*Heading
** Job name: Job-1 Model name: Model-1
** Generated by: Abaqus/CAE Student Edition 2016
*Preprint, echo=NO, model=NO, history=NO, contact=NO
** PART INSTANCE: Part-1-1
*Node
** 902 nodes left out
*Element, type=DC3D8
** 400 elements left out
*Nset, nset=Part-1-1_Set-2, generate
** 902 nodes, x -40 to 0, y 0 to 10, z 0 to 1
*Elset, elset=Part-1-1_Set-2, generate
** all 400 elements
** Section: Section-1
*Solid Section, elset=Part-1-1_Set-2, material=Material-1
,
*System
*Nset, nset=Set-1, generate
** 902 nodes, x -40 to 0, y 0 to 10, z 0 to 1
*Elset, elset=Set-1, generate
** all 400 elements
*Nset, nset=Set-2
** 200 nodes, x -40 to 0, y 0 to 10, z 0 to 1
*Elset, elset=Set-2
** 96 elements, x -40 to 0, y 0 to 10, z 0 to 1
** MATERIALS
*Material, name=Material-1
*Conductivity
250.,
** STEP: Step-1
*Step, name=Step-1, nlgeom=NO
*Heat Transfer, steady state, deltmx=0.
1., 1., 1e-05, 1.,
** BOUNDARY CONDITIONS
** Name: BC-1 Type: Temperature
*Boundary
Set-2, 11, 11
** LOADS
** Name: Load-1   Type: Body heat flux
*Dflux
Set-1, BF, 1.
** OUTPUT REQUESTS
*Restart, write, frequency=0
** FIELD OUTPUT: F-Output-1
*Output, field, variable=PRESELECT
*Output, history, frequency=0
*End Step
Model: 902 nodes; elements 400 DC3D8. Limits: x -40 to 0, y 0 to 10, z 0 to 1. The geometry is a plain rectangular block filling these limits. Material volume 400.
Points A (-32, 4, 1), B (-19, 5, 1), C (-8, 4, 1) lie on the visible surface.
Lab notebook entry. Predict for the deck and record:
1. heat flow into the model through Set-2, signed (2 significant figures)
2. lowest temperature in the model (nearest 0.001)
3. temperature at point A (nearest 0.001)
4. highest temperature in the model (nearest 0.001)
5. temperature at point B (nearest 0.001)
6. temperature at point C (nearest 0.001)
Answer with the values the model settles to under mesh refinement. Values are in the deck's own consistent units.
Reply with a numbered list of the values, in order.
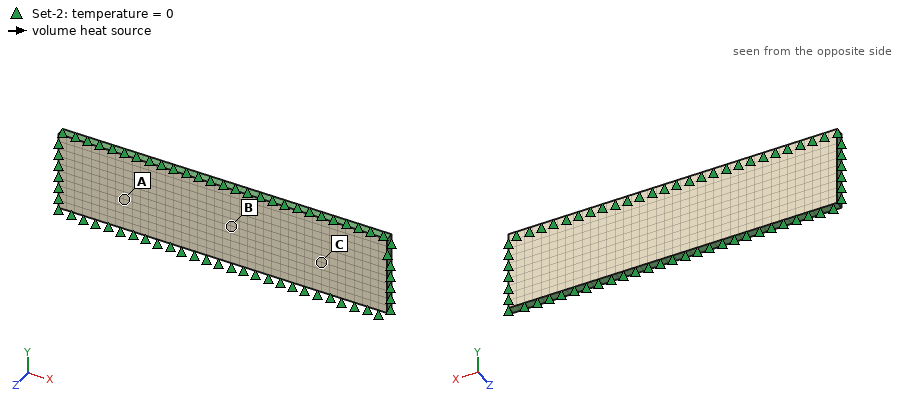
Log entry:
1. -390
2. 0.000
3. 0.044
4. 0.050
5. 0.050
6. 0.044
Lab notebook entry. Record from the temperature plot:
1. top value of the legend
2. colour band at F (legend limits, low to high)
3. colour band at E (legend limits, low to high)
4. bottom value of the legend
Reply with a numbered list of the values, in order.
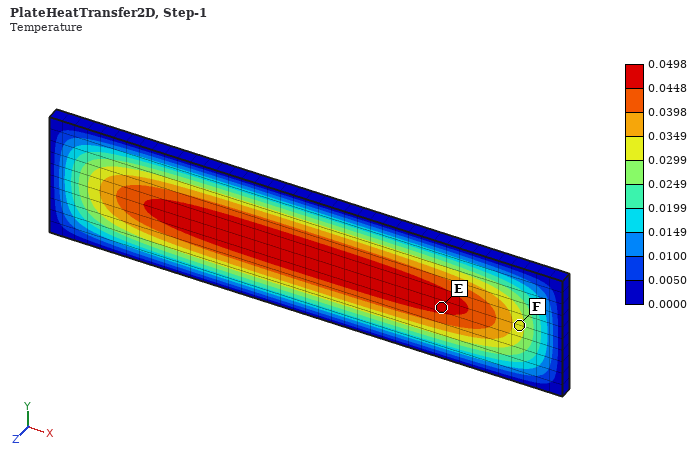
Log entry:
1. 0.0498
2. 0.0299 to 0.0349
3. 0.0448 to 0.0498
4. 0.0000
